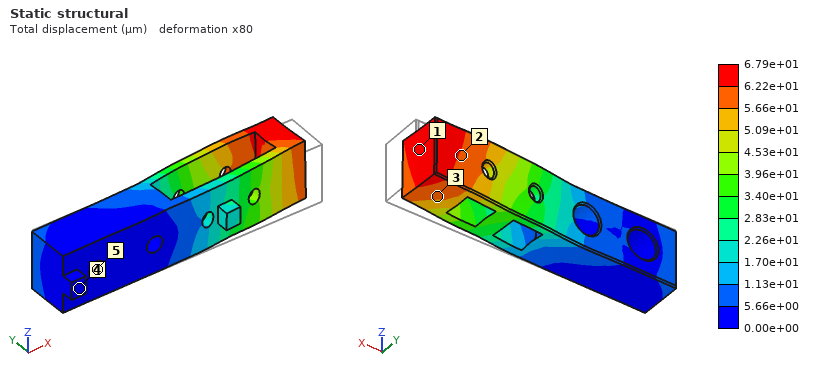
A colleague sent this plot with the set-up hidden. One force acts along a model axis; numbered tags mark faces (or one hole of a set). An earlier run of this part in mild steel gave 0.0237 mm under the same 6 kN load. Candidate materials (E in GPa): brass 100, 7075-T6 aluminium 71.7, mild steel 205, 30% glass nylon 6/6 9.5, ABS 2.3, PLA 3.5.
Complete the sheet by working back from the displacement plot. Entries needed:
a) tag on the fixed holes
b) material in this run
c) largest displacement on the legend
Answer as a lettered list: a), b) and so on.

a) 5
b) 7075-T6 aluminium
c) 6.79e+01 µm
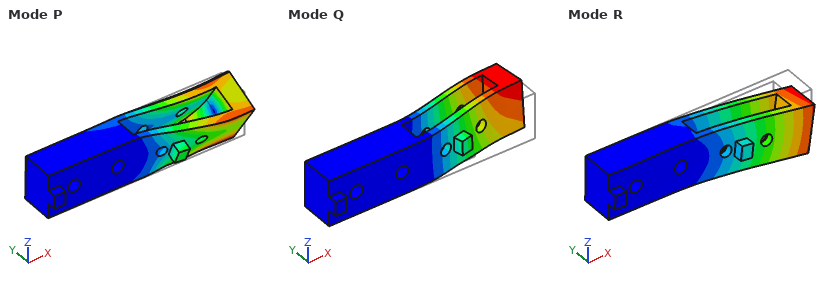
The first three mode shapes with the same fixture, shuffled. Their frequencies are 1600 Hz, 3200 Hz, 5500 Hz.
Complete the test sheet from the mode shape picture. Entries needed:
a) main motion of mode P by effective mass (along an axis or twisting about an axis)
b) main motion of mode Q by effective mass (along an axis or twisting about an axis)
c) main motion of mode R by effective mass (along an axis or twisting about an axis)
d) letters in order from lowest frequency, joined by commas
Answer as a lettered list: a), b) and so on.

a) twisting about X
b) along Y
c) along Z
d) Q, R, P
